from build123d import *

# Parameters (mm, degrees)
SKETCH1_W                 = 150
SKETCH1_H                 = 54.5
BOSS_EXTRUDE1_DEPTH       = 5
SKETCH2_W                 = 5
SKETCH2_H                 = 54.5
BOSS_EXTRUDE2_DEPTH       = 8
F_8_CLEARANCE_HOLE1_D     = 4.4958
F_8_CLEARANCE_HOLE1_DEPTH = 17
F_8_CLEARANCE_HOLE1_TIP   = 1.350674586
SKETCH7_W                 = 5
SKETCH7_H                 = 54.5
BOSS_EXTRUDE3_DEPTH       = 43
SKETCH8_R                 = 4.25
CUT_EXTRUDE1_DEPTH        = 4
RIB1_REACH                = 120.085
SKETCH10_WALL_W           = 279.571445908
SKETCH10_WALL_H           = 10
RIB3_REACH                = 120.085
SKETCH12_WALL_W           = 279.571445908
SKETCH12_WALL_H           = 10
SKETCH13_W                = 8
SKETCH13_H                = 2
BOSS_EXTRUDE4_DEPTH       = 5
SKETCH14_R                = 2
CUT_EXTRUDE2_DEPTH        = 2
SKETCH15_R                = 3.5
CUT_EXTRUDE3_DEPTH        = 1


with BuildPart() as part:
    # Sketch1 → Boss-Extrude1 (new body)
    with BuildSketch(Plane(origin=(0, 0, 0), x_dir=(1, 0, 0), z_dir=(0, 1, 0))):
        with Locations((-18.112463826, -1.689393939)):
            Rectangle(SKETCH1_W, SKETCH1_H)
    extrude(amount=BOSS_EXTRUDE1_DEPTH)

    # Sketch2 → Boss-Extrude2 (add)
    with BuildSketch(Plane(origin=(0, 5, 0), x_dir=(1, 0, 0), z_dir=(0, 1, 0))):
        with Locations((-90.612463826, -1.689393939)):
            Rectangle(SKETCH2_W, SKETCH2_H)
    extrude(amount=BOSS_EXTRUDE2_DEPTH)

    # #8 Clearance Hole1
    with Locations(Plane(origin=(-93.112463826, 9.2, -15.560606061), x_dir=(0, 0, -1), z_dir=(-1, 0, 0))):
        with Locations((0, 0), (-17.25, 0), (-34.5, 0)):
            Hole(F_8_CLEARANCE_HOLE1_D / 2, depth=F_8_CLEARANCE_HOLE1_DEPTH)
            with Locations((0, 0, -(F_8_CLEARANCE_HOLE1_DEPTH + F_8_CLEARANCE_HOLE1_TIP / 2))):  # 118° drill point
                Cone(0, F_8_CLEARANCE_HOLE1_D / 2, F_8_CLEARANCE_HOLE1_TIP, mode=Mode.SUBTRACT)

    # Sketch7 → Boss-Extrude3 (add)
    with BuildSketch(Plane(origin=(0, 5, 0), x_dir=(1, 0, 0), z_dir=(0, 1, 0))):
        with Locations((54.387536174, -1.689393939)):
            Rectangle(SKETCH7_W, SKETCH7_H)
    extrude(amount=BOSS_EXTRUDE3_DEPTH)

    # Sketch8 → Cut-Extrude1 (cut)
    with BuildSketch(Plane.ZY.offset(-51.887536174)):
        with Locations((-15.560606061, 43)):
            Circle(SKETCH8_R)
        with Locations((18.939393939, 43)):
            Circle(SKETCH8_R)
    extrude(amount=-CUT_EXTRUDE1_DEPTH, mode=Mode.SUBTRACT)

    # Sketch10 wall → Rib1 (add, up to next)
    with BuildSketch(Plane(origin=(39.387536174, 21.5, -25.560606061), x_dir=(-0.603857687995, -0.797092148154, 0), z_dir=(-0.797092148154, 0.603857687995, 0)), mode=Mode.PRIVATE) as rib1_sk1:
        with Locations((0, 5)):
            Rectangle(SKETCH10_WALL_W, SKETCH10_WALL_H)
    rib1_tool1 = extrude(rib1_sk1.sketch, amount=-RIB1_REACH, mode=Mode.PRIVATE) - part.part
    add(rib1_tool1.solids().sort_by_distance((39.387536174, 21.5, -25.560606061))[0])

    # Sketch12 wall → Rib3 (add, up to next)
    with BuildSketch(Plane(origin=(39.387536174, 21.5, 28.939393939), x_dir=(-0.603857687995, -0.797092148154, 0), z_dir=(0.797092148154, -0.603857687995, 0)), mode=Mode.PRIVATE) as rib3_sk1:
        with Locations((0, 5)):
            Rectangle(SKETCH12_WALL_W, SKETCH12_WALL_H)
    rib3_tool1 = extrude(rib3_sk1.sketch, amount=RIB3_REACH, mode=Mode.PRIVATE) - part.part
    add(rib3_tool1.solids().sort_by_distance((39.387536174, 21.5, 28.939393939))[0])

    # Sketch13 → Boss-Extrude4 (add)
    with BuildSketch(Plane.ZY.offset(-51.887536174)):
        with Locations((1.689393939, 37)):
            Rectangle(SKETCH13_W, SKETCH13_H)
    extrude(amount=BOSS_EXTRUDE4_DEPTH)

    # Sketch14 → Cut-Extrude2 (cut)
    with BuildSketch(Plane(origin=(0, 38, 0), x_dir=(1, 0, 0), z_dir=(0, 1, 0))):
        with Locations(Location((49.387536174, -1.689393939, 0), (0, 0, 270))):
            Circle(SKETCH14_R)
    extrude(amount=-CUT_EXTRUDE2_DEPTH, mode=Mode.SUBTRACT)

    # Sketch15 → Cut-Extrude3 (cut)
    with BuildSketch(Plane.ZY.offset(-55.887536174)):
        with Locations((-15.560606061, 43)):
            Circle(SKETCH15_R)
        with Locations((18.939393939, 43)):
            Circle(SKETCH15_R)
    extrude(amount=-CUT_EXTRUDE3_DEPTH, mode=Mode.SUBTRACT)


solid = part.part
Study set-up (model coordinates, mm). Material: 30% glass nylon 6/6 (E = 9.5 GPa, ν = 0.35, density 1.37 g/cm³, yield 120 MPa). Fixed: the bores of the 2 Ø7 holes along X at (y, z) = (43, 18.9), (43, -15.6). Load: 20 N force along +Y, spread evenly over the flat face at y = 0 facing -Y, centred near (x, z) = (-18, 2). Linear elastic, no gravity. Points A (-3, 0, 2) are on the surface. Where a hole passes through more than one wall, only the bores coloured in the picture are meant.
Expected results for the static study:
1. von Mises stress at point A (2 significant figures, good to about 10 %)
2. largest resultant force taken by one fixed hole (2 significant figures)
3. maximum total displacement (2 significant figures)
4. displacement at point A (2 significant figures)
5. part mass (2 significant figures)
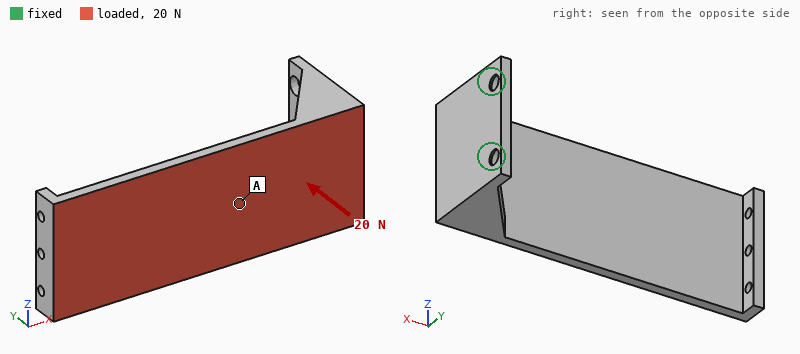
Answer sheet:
2.3 MPa
21 N
1.9 mm
0.62 mm
85 g
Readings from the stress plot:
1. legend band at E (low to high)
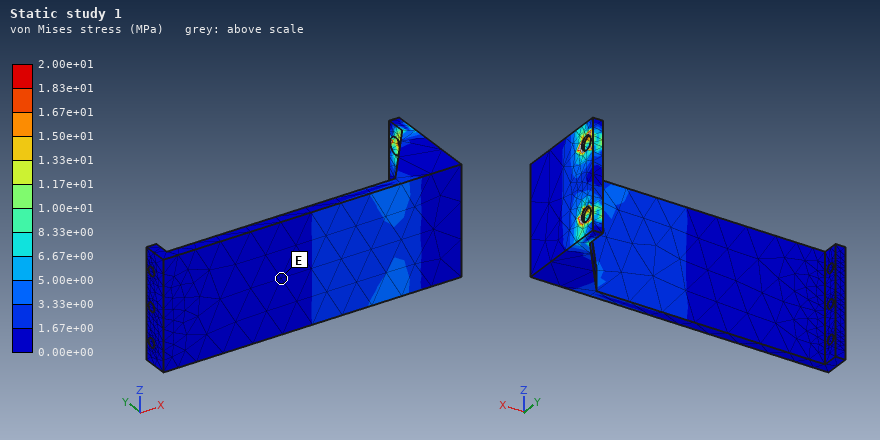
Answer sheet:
0.00e+00 to 1.67e+00 MPa
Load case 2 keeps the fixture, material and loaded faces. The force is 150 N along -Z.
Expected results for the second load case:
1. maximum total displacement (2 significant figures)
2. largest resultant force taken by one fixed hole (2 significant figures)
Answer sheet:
2.0 mm
350 N
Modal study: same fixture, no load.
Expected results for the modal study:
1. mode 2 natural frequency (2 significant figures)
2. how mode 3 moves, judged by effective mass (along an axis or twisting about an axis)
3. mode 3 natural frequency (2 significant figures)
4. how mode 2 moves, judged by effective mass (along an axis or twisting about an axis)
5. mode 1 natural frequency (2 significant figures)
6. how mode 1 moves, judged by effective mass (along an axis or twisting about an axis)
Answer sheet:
210 Hz
along X
310 Hz
along Z
78 Hz
along Y
